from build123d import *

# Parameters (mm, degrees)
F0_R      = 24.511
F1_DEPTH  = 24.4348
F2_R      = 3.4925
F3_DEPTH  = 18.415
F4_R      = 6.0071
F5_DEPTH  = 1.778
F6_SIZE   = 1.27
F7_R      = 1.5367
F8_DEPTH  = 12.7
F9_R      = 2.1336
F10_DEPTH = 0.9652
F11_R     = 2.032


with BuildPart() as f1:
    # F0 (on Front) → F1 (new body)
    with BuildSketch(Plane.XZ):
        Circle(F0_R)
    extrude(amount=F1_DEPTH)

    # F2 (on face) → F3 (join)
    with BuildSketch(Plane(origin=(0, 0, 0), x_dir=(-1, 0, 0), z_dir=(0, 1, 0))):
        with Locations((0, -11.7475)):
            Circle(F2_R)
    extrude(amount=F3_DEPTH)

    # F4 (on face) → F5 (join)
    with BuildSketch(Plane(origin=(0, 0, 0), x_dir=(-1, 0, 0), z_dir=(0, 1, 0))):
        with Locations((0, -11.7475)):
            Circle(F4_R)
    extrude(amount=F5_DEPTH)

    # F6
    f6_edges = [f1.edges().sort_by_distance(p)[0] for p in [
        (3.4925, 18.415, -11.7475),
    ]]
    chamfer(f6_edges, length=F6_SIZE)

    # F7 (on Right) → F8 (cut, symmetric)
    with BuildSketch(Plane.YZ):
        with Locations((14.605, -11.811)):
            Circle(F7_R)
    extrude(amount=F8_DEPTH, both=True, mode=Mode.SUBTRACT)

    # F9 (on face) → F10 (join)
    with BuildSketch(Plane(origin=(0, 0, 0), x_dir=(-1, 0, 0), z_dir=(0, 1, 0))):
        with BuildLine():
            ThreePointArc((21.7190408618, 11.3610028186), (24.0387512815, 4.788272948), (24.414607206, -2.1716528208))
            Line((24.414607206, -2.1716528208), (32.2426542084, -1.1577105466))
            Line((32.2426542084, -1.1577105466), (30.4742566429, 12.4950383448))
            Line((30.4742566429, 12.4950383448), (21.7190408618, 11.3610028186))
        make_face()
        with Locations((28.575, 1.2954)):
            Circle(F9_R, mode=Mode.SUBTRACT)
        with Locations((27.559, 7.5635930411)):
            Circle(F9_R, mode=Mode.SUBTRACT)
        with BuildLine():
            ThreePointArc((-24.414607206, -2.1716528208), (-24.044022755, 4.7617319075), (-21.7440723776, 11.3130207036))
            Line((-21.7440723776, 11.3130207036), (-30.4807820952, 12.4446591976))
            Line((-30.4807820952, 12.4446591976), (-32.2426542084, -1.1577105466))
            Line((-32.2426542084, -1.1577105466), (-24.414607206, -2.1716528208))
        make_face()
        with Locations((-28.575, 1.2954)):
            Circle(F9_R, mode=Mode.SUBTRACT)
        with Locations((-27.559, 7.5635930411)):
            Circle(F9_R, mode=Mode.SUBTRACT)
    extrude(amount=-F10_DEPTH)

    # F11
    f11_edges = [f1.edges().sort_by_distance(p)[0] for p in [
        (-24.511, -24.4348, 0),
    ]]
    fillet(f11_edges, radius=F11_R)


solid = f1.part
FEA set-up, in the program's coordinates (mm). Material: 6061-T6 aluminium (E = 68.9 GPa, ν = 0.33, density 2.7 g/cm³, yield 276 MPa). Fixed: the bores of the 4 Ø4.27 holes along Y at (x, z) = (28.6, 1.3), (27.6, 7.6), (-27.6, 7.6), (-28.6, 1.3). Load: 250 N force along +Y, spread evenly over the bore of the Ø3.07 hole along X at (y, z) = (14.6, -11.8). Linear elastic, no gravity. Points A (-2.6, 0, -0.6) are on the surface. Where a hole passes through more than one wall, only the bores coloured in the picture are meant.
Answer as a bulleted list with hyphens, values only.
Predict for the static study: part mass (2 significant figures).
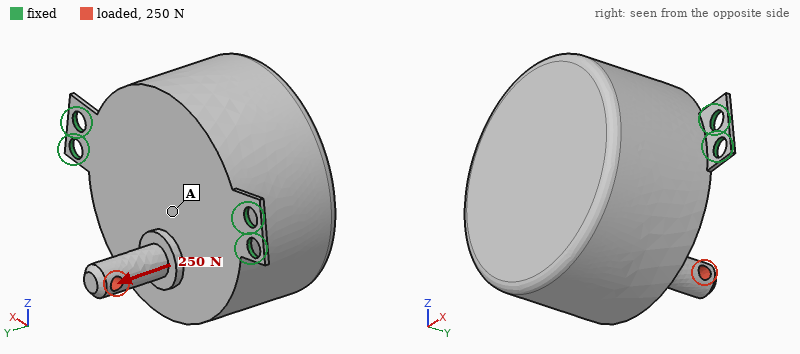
- 130 g
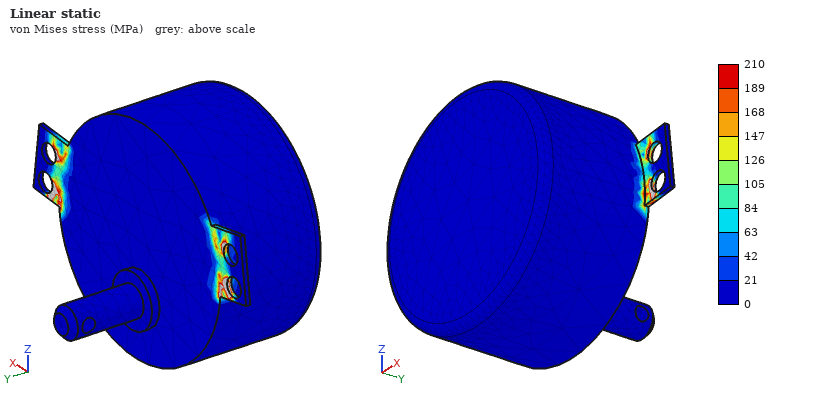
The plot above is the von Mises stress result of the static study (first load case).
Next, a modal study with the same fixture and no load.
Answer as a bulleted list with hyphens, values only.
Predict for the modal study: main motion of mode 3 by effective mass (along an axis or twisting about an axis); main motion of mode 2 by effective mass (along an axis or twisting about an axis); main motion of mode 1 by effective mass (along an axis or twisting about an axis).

- along X
- along Y
- along Z
